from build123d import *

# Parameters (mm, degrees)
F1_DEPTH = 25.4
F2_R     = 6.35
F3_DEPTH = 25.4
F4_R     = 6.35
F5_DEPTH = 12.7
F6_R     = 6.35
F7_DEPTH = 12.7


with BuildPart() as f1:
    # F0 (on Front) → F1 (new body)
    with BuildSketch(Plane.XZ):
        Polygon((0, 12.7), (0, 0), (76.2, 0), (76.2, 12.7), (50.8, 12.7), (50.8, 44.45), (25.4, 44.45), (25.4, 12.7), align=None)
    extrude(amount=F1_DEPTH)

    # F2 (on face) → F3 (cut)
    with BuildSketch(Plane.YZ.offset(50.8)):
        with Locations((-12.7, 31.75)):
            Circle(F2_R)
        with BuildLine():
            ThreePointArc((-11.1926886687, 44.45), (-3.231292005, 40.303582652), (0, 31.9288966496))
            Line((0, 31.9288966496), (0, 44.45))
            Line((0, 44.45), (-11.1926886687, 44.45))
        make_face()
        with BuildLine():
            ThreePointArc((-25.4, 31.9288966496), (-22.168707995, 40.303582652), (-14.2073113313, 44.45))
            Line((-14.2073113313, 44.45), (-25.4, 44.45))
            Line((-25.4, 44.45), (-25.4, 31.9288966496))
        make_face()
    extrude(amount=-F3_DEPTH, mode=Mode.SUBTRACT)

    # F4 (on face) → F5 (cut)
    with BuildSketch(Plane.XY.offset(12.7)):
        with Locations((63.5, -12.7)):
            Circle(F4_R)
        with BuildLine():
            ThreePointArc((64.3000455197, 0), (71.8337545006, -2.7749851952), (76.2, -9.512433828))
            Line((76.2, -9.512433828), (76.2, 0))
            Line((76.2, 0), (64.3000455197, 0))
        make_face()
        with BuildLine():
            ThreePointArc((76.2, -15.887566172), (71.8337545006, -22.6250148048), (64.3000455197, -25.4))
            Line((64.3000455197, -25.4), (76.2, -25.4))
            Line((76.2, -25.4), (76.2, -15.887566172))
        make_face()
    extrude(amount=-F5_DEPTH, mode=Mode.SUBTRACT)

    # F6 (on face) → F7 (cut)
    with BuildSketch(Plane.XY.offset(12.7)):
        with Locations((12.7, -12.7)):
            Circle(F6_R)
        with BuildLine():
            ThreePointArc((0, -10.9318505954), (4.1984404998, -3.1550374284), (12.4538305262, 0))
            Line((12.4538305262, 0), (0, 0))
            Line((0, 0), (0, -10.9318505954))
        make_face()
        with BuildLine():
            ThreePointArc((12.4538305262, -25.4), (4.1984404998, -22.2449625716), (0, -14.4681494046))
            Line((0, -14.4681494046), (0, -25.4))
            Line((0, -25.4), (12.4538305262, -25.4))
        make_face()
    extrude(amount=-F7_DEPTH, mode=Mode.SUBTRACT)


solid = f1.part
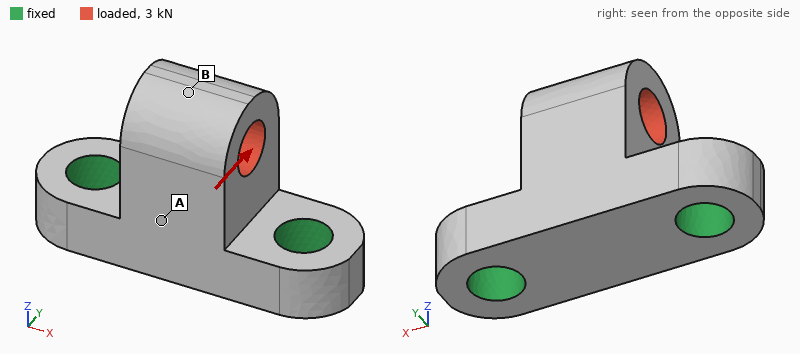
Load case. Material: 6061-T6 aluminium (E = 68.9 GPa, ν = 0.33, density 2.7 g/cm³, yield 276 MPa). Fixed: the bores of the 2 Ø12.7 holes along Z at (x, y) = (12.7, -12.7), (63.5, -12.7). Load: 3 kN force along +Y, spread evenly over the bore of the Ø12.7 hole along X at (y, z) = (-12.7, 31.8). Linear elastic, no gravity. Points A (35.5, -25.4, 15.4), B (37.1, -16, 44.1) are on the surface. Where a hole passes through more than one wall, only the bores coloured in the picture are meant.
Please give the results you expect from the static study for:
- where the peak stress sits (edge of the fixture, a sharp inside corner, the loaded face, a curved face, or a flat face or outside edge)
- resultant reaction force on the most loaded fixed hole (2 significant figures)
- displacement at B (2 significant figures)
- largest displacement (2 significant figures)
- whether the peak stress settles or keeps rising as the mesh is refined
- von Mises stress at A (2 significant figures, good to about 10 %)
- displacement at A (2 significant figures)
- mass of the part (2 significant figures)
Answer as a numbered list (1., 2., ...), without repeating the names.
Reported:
1. edge of the fixture
2. 1.5 kN
3. 66 µm
4. 66 µm
5. keeps rising
6. 13 MPa
7. 24 µm
8. 95 g
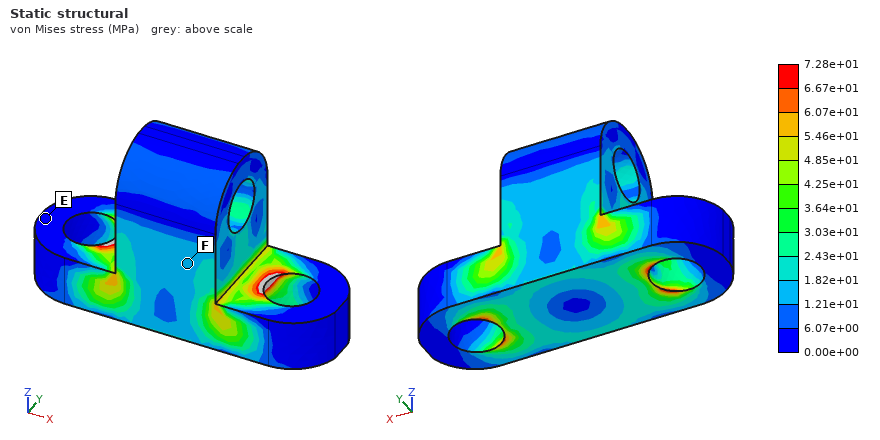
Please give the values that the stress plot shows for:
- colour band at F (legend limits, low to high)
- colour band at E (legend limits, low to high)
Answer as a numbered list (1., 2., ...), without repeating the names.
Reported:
1. 1.21e+01 to 1.82e+01 MPa
2. 0.00e+00 to 6.07e+00 MPa
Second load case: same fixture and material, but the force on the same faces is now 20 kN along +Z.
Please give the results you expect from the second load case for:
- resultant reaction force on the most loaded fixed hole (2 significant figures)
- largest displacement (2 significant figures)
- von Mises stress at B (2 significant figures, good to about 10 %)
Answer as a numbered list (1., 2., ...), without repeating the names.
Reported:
1. 10 kN
2. 46 µm
3. 34 MPa
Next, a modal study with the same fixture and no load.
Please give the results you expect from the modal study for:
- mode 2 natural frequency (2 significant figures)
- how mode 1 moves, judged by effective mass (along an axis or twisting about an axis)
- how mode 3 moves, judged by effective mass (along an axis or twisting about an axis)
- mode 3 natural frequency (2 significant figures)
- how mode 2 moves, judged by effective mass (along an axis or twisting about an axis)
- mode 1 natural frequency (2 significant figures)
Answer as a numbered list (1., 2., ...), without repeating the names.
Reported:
1. 12 kHz
2. along Y
3. along Z
4. 17 kHz
5. along X
6. 6900 Hz
